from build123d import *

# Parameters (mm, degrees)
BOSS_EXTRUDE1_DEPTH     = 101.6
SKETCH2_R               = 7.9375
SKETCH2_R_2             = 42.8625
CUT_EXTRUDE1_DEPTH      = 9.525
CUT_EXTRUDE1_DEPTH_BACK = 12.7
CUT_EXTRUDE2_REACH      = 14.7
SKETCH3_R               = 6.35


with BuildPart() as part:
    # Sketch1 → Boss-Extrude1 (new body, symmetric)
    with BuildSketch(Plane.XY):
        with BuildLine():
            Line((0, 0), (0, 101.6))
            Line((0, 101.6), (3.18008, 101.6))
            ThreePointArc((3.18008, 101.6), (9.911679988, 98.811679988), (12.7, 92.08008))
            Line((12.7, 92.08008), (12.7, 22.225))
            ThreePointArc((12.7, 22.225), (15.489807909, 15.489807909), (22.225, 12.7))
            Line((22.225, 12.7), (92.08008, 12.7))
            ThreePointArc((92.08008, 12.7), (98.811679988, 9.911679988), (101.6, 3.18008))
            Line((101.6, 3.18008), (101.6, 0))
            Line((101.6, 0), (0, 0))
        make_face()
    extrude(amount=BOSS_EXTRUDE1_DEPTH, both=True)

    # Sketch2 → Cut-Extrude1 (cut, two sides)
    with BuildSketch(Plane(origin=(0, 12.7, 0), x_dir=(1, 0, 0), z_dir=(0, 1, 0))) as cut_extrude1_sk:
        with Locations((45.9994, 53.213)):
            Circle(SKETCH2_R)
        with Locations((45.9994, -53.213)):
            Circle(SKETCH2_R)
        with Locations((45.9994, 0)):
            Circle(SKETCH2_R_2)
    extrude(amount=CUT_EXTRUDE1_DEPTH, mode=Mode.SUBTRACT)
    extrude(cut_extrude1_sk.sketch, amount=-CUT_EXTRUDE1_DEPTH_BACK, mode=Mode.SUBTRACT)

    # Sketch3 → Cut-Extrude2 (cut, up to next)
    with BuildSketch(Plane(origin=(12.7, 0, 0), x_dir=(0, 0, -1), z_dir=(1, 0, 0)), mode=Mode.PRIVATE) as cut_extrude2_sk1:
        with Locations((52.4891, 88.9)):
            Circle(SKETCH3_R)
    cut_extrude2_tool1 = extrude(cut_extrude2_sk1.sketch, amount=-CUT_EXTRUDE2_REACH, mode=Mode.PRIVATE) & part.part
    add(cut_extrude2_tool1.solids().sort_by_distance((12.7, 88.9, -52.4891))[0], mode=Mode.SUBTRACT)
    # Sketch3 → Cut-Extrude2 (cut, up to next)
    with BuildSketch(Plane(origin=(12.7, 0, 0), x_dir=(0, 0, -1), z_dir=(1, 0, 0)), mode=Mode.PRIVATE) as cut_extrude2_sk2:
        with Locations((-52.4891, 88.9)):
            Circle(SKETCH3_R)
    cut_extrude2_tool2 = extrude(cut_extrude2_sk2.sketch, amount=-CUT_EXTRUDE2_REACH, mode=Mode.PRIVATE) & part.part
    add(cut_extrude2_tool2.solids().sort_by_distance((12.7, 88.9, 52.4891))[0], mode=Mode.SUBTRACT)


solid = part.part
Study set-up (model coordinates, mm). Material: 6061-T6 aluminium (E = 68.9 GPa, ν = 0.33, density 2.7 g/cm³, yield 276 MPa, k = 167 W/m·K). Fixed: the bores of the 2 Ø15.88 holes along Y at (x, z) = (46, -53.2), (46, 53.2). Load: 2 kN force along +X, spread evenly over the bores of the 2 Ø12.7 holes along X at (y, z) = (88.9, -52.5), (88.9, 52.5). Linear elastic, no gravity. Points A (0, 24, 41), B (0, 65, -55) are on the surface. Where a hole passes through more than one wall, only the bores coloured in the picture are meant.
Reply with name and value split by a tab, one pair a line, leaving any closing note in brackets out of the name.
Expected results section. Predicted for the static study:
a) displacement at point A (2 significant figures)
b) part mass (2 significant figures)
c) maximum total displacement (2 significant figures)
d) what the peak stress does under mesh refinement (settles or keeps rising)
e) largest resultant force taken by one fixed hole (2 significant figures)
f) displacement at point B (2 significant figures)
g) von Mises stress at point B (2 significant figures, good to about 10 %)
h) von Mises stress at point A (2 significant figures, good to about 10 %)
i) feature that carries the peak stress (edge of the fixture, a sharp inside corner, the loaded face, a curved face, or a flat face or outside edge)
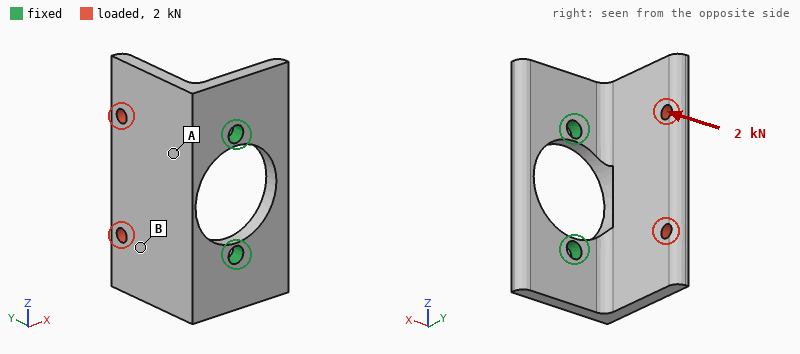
displacement at point A	0.14 mm
part mass	1.1 kg
maximum total displacement	0.55 mm
what the peak stress does under mesh refinement	keeps rising
largest resultant force taken by one fixed hole	1.0 kN
displacement at point B	0.32 mm
von Mises stress at point B	11 MPa
von Mises stress at point A	25 MPa
feature that carries the peak stress	edge of the fixture
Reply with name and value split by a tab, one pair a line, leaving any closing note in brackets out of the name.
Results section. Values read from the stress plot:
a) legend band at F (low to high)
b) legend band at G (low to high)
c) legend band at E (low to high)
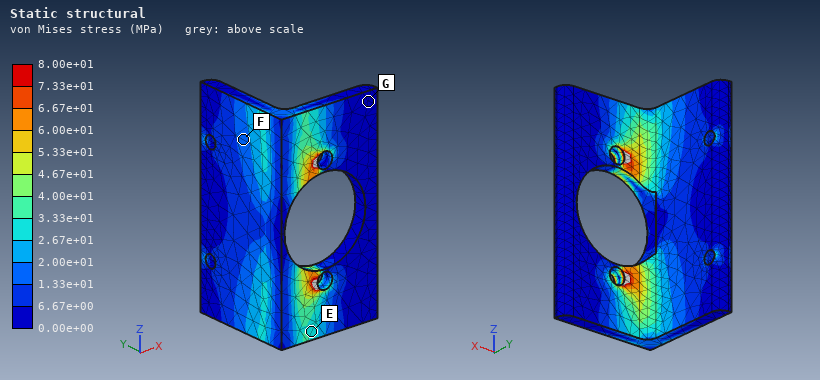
legend band at F	1.33e+01 to 2.00e+01 MPa
legend band at G	0.00e+00 to 6.67e+00 MPa
legend band at E	2.67e+01 to 3.33e+01 MPa
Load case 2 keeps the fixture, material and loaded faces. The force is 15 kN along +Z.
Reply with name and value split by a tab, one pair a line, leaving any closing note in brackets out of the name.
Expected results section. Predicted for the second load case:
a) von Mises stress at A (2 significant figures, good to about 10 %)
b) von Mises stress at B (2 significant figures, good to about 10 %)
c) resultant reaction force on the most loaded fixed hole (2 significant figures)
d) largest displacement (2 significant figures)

von Mises stress at A	37 MPa
von Mises stress at B	22 MPa
resultant reaction force on the most loaded fixed hole	12 kN
largest displacement	0.56 mm
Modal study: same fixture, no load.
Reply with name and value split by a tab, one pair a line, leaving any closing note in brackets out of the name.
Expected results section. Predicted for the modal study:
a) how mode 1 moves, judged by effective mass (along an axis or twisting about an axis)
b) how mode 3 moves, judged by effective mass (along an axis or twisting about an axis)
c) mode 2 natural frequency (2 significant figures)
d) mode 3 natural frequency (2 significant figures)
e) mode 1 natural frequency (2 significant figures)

how mode 1 moves, judged by effective mass	along X
how mode 3 moves, judged by effective mass	along Z
mode 2 natural frequency	1100 Hz
mode 3 natural frequency	2000 Hz
mode 1 natural frequency	630 Hz
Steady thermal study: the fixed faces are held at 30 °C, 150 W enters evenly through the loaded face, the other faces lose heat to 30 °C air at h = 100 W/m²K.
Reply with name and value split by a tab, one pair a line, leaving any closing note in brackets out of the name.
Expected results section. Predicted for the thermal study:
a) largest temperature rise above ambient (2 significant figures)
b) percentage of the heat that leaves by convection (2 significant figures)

largest temperature rise above ambient	40 K
percentage of the heat that leaves by convection	61 %
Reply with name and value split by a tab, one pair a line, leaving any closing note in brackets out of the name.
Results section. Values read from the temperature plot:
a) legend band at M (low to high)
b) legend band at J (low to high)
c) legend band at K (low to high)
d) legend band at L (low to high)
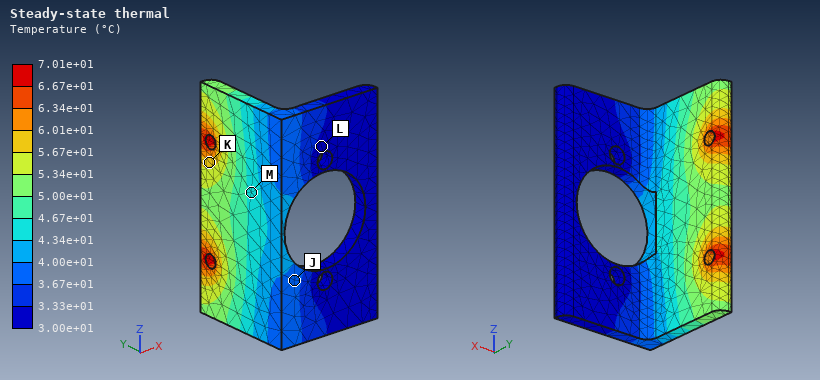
legend band at M	4.34e+01 to 4.67e+01 °C
legend band at J	3.67e+01 to 4.00e+01 °C
legend band at K	5.67e+01 to 6.01e+01 °C
legend band at L	3.00e+01 to 3.33e+01 °C
